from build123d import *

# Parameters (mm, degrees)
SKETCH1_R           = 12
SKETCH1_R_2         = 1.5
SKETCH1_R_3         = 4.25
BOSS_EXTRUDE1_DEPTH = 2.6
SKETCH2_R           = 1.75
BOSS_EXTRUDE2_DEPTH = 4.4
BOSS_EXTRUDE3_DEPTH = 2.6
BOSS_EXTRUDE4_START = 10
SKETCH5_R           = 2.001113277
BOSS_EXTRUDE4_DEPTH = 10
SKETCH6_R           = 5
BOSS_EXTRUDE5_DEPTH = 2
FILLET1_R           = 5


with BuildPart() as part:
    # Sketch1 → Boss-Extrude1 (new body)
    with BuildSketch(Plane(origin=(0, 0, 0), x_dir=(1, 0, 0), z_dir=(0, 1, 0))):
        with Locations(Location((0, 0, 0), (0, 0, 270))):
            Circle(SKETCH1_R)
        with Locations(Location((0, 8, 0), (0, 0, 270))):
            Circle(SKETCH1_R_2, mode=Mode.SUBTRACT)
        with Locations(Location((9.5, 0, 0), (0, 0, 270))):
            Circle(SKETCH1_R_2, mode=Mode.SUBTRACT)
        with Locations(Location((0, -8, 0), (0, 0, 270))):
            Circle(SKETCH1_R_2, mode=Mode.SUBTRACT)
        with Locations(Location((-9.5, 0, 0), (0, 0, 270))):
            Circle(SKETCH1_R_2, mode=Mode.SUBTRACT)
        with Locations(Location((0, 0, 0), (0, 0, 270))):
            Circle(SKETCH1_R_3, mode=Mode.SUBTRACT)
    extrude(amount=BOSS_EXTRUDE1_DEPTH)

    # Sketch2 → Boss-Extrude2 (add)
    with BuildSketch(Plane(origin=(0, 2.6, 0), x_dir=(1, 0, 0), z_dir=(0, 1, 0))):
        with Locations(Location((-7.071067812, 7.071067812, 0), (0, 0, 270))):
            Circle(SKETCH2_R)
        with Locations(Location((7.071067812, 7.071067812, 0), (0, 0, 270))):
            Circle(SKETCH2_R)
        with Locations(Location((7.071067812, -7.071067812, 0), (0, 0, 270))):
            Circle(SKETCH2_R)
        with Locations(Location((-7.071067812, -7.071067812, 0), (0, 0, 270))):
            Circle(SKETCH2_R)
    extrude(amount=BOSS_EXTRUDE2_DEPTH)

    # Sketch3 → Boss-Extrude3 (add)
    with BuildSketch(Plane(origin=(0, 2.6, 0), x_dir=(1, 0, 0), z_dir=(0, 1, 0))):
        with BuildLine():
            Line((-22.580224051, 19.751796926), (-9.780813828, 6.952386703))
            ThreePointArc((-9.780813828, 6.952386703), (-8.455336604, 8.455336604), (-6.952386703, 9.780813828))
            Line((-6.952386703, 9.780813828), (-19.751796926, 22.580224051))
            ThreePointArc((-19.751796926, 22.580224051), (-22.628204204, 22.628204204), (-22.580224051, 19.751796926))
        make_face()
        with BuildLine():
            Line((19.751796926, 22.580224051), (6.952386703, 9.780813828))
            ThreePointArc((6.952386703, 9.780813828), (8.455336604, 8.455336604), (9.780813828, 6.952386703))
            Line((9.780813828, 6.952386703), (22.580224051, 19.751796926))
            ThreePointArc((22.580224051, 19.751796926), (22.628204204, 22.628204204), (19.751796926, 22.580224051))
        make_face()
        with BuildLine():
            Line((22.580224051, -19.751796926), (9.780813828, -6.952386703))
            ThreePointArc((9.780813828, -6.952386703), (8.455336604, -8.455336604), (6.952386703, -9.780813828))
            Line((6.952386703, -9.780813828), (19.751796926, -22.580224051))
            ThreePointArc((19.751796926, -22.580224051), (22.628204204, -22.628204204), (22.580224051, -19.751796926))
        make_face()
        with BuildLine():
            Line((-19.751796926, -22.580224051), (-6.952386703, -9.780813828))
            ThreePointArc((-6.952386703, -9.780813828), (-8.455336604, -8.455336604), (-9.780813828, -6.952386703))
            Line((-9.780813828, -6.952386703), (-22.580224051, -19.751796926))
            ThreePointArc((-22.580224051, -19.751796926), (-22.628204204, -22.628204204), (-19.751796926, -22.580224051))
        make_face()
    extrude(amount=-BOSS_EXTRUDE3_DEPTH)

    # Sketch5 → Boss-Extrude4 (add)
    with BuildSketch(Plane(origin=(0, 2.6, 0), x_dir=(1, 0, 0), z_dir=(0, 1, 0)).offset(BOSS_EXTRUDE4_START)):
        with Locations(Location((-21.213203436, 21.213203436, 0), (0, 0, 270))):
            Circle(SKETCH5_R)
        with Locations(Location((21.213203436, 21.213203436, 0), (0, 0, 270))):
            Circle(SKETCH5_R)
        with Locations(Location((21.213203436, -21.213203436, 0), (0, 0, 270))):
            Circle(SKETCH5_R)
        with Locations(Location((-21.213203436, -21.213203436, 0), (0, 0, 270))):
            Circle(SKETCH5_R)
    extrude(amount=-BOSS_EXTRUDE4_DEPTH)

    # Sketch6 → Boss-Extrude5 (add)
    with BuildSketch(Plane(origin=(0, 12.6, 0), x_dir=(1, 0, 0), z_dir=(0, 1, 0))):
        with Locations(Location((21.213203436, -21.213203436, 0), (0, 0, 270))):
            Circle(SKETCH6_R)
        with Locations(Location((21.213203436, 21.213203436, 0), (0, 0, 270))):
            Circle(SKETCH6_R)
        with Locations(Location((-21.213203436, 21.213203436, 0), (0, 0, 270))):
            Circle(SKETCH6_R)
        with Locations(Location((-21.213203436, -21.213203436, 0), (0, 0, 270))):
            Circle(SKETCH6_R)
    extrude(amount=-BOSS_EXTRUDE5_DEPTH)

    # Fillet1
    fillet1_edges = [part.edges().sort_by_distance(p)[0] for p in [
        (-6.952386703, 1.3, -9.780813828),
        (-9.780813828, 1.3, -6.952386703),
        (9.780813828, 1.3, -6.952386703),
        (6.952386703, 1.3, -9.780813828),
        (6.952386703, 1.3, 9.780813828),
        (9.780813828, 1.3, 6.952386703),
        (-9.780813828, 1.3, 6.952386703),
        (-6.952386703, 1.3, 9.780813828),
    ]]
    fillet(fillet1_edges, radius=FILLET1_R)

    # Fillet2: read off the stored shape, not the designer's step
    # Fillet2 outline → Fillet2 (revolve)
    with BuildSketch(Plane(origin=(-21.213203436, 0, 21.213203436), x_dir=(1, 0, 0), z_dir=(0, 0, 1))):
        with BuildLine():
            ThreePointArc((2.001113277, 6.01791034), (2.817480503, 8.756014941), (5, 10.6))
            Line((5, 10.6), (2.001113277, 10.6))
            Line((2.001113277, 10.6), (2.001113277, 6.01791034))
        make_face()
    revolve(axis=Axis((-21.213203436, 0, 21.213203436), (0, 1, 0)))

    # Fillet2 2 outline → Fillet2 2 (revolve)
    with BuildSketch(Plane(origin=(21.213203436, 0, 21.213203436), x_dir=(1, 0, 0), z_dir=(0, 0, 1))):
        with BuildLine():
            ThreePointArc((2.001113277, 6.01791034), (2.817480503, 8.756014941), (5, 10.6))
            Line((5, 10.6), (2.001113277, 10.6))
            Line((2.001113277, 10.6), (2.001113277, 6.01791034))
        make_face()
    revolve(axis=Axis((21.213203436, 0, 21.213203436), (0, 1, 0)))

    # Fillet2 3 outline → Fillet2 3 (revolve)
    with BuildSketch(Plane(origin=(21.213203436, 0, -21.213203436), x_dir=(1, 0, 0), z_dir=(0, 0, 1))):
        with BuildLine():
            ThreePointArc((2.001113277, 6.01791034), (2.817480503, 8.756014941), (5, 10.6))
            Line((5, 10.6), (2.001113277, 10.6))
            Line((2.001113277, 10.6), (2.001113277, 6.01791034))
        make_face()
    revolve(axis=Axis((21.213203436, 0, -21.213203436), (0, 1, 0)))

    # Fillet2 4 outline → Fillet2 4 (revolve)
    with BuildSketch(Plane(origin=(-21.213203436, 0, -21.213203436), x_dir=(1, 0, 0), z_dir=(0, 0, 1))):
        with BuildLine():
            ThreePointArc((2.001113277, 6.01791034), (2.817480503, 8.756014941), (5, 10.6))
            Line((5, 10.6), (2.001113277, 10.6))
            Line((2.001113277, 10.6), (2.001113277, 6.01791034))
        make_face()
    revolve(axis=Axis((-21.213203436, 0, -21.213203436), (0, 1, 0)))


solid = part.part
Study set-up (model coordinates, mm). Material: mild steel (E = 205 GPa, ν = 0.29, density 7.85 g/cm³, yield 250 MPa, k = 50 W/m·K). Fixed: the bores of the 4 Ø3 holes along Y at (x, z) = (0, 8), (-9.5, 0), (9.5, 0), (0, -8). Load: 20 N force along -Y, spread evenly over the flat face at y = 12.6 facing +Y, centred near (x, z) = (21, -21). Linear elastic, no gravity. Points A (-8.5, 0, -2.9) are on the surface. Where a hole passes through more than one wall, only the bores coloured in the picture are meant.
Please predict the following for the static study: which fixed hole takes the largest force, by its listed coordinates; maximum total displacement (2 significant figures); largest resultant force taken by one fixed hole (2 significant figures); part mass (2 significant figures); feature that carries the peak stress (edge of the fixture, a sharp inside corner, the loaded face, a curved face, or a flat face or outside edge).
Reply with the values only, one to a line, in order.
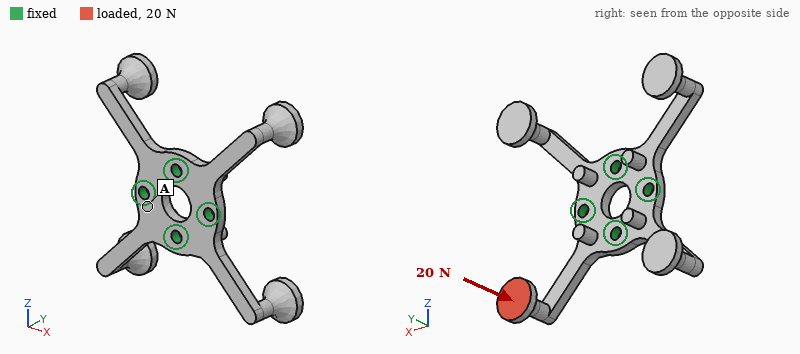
(9.5, 0)
74 µm
15 N
26 g
a curved face
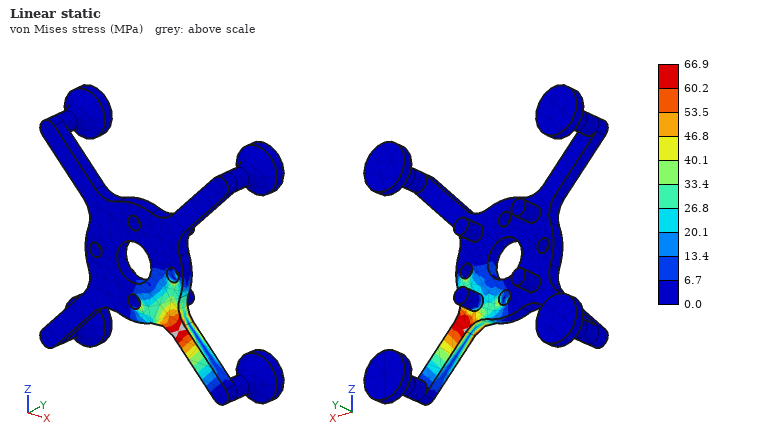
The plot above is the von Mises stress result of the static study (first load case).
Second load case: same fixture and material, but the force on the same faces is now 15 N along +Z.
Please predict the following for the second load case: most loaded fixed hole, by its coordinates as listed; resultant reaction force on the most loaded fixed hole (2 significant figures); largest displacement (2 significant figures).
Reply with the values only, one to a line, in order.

(9.5, 0)
29 N
51 µm
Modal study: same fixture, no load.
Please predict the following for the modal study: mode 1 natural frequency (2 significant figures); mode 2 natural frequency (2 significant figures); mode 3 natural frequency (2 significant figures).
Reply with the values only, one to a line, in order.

1600 Hz
1600 Hz
1600 Hz
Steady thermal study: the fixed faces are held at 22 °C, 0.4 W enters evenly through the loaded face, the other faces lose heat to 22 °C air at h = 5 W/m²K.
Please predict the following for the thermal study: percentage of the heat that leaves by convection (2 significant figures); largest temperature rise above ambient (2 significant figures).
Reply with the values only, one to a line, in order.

7.7 %
18 K
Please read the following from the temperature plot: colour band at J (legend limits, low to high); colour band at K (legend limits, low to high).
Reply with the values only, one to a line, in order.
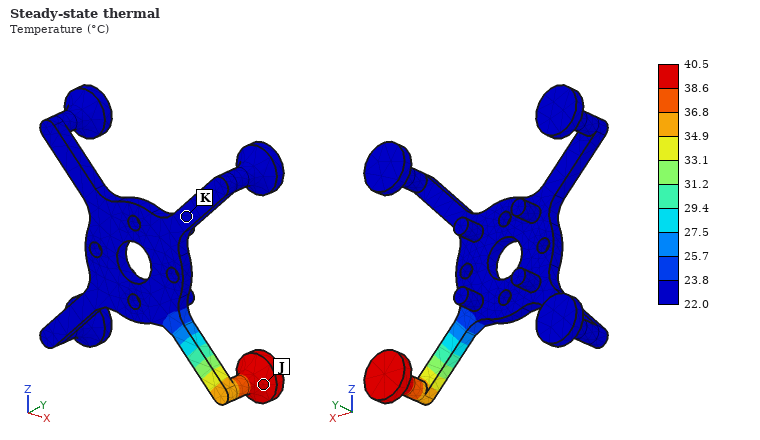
38.6 to 40.5 °C
22.0 to 23.8 °C
